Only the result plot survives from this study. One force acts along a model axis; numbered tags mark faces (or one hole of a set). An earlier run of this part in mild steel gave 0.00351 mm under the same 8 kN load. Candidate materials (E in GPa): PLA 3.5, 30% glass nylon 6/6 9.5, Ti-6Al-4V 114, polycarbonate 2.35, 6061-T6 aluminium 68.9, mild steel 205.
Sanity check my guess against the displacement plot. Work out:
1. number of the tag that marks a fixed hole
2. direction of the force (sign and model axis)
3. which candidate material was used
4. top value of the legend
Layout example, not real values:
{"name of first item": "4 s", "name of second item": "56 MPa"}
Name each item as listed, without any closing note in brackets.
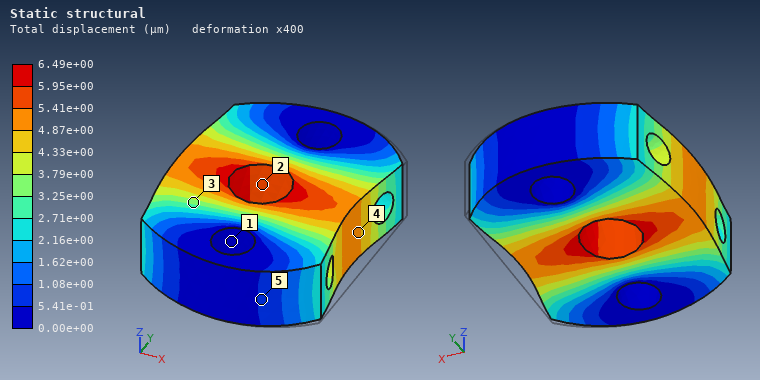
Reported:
{"number of the tag that marks a fixed hole": "1", "direction of the force": "-X", "which candidate material was used": "Ti-6Al-4V", "top value of the legend": "6.49e+00 µm"}
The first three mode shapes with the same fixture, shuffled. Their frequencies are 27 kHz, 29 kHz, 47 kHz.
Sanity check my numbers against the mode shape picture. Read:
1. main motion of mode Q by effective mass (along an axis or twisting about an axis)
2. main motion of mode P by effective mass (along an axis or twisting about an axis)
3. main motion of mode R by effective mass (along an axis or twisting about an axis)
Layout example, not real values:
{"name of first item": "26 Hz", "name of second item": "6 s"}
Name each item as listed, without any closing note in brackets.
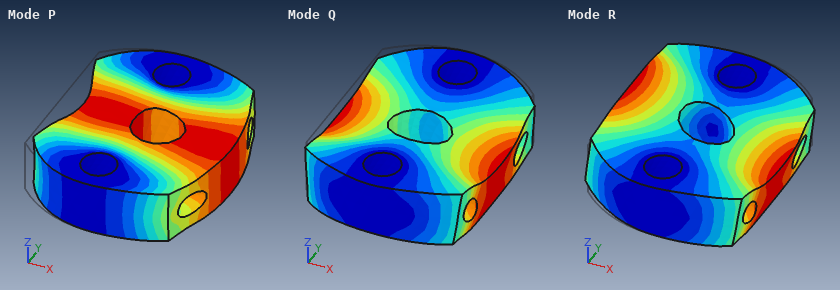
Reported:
{"main motion of mode Q by effective mass": "along Z", "main motion of mode P by effective mass": "along X", "main motion of mode R by effective mass": "twisting about Y"}
